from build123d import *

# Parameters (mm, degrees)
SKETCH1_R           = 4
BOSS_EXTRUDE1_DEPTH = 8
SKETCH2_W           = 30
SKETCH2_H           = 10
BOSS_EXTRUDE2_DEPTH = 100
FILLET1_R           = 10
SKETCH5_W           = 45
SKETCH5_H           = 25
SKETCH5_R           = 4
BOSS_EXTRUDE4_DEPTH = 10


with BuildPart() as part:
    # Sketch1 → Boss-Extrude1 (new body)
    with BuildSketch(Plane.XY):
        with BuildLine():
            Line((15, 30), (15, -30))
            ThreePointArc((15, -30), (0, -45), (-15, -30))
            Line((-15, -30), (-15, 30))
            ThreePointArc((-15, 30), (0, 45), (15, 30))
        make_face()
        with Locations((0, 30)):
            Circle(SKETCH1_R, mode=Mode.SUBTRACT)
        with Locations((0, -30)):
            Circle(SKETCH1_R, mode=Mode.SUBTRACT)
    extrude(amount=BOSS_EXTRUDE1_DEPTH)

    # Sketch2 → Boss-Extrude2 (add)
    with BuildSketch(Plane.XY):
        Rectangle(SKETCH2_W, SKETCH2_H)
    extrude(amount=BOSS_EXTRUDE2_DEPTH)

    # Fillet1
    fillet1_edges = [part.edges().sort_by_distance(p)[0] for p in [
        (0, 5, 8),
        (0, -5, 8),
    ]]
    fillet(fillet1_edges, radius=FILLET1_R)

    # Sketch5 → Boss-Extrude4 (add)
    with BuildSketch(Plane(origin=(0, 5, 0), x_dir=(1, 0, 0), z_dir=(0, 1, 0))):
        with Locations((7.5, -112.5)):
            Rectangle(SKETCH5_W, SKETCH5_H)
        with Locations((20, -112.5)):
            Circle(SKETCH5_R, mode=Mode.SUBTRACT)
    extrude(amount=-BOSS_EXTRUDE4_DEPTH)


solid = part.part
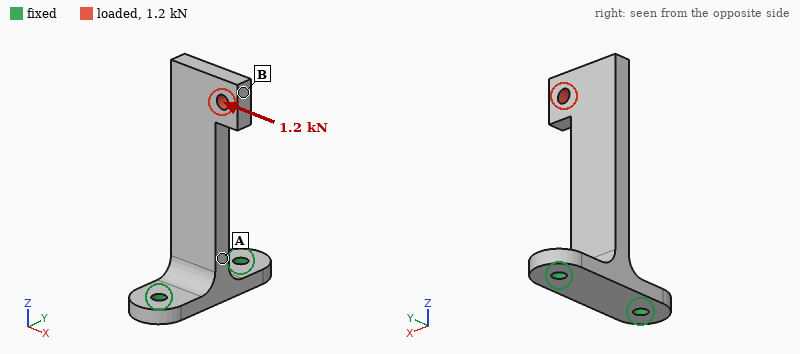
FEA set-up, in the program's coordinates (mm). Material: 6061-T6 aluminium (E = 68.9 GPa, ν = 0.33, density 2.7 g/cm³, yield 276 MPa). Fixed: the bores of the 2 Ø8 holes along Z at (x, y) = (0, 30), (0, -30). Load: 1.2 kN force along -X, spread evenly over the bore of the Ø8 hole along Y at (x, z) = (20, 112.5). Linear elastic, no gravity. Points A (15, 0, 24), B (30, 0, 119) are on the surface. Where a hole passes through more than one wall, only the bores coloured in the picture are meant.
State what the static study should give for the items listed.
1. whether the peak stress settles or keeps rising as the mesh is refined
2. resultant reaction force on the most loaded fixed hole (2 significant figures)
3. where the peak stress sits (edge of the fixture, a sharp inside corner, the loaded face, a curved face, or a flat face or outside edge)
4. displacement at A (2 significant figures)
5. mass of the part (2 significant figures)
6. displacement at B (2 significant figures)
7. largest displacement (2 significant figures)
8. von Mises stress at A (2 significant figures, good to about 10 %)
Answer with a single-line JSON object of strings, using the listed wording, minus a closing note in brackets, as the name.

{"whether the peak stress settles or keeps rising as the mesh is refined": "keeps rising", "resultant reaction force on the most loaded fixed hole": "600 N", "where the peak stress sits": "edge of the fixture", "displacement at A": "0.26 mm", "mass of the part": "160 g", "displacement at B": "1.5 mm", "largest displacement": "1.5 mm", "von Mises stress at A": "72 MPa"}
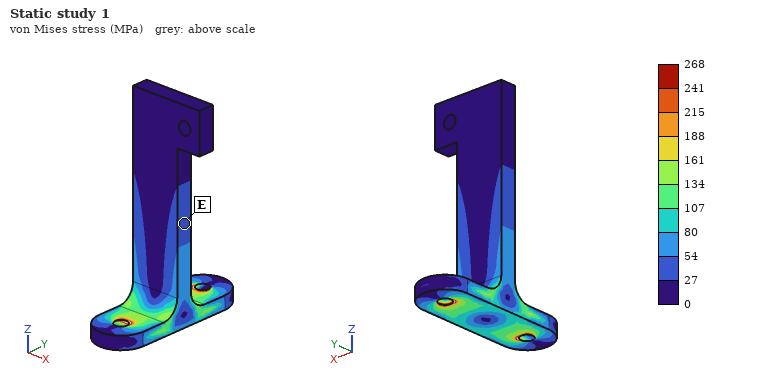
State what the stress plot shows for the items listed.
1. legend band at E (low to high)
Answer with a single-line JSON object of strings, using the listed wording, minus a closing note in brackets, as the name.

{"legend band at E": "27 to 54 MPa"}
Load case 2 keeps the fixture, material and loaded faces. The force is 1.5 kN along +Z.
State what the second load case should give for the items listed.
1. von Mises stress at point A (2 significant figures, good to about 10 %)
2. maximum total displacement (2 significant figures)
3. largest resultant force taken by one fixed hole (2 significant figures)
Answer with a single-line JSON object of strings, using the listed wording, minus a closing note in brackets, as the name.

{"von Mises stress at point A": "25 MPa", "maximum total displacement": "0.41 mm", "largest resultant force taken by one fixed hole": "820 N"}
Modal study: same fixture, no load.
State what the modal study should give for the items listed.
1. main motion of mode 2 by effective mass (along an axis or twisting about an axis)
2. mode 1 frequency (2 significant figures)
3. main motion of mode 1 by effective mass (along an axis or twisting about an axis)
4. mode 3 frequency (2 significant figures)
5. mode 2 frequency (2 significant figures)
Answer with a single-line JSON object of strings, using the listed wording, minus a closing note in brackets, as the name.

{"main motion of mode 2 by effective mass": "along X", "mode 1 frequency": "530 Hz", "main motion of mode 1 by effective mass": "along Y", "mode 3 frequency": "2700 Hz", "mode 2 frequency": "690 Hz"}
